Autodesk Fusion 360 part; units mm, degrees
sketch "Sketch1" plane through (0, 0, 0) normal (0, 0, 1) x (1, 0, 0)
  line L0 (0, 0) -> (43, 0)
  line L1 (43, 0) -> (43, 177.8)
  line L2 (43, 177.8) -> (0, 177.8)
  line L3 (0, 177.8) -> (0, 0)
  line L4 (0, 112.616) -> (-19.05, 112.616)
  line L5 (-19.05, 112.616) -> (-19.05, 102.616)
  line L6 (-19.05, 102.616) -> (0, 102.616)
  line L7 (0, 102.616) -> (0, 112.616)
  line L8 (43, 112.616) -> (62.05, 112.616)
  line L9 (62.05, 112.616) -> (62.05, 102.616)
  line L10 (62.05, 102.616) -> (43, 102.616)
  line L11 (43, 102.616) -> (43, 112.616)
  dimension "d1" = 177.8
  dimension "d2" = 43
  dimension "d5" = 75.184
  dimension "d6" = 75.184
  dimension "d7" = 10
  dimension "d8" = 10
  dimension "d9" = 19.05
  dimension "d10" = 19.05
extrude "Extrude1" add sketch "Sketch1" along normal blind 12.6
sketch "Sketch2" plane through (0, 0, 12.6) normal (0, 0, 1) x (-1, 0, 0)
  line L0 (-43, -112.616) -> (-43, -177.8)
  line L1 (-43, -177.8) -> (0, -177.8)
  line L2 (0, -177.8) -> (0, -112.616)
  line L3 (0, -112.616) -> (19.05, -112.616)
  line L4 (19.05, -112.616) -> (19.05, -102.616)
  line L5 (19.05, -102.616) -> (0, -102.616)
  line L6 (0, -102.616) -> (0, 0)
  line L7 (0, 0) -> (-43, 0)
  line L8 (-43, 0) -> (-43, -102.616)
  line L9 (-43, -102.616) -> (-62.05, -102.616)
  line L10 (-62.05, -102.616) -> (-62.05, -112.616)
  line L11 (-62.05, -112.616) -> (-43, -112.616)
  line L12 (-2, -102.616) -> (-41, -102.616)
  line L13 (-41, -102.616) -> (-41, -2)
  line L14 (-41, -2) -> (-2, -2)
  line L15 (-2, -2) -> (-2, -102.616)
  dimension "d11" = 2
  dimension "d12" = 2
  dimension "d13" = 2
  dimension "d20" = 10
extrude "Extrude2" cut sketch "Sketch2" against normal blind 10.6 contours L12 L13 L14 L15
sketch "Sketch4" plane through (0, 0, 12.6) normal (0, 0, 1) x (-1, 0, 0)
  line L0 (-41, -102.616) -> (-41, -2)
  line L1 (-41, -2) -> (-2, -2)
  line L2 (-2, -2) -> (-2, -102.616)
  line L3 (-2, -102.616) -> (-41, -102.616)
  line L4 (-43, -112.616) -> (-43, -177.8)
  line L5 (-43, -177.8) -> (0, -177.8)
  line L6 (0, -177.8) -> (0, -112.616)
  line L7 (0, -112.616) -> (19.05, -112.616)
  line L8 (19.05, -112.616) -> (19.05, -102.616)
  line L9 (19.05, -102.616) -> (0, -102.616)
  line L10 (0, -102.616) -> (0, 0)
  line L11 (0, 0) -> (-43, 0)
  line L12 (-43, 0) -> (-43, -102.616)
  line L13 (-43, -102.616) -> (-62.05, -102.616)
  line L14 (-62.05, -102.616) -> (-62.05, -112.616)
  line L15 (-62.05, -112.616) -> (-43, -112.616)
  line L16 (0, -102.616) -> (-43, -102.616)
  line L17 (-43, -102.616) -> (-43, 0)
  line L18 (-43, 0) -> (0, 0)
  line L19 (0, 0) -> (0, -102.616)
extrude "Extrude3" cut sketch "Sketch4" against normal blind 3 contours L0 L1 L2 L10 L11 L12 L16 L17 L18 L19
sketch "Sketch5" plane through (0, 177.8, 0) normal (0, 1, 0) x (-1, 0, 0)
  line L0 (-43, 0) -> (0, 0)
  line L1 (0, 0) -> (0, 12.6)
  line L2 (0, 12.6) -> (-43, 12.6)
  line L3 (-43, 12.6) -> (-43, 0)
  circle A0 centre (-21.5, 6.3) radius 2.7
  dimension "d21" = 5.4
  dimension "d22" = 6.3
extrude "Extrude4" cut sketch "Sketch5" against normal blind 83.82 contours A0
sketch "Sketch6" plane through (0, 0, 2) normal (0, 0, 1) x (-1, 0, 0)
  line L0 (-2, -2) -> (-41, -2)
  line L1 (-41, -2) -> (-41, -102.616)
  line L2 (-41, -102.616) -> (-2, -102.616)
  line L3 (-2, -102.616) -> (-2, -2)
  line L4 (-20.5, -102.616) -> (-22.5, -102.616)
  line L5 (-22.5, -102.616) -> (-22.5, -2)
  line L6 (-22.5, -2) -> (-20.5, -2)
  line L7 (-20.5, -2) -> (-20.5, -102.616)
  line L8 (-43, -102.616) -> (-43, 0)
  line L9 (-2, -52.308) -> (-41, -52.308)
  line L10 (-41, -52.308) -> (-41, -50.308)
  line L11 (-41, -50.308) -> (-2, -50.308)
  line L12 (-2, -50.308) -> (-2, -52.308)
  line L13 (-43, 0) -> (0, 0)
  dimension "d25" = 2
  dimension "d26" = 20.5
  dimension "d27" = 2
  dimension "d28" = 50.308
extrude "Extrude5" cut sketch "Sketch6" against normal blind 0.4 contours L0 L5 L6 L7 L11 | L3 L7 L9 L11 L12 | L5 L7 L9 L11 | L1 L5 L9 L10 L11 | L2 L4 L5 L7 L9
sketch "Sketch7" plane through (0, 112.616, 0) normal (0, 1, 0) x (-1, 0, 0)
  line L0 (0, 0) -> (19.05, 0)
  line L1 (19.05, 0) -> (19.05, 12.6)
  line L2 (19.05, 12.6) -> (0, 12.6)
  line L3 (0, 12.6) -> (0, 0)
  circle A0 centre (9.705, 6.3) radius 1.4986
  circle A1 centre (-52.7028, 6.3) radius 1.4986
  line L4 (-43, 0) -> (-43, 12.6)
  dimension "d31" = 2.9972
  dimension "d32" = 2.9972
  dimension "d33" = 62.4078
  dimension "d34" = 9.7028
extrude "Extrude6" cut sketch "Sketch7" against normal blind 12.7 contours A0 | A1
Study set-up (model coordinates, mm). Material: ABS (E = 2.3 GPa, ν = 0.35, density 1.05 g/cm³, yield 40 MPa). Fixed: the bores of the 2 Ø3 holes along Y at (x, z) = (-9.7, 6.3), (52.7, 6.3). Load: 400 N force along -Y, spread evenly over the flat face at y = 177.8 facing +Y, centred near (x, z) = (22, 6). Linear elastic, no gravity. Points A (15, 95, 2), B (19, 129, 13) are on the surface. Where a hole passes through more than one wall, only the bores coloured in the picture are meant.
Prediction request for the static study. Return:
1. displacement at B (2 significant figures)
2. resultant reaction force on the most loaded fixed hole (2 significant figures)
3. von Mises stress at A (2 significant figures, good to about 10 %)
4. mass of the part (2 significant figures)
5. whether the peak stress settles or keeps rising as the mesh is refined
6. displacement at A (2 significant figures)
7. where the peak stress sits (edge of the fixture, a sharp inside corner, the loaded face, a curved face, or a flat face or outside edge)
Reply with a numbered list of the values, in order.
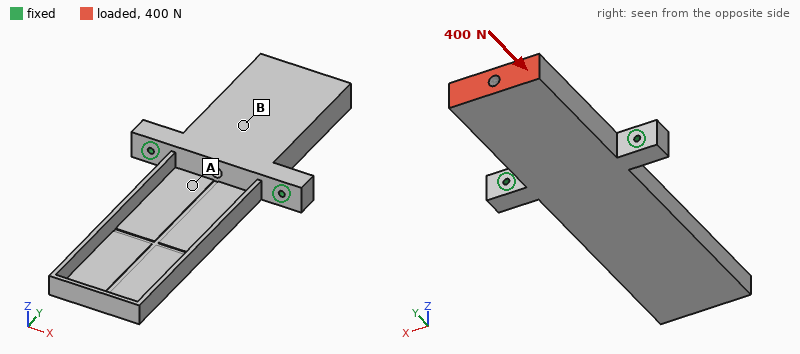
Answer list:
1. 0.060 mm
2. 210 N
3. 1.1 MPa
4. 59 g
5. keeps rising
6. 0.050 mm
7. edge of the fixture
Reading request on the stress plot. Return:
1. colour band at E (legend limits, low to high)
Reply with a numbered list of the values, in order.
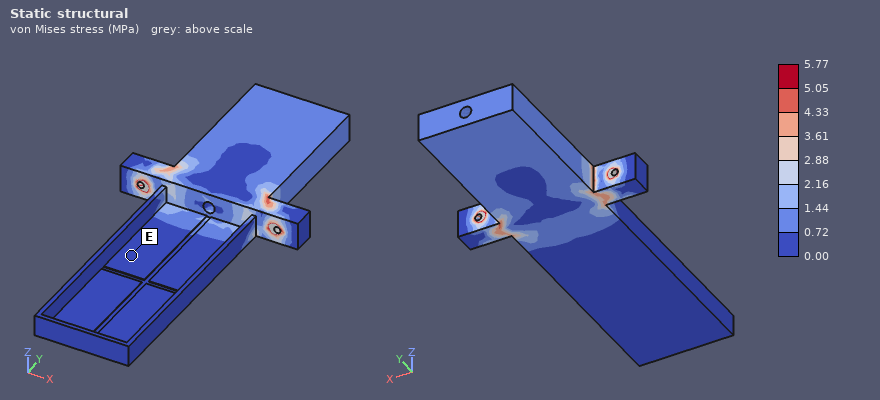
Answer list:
1. 0.00 to 0.72 MPa
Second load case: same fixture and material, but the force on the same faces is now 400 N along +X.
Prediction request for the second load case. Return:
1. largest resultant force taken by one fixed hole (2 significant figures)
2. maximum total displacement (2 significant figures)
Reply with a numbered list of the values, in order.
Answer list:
1. 570 N
2. 0.65 mm
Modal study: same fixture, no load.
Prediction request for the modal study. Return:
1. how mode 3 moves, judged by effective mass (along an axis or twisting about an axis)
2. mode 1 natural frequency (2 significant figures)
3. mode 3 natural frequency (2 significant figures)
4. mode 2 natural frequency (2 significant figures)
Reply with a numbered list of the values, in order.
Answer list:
1. along Z
2. 150 Hz
3. 320 Hz
4. 280 Hz
